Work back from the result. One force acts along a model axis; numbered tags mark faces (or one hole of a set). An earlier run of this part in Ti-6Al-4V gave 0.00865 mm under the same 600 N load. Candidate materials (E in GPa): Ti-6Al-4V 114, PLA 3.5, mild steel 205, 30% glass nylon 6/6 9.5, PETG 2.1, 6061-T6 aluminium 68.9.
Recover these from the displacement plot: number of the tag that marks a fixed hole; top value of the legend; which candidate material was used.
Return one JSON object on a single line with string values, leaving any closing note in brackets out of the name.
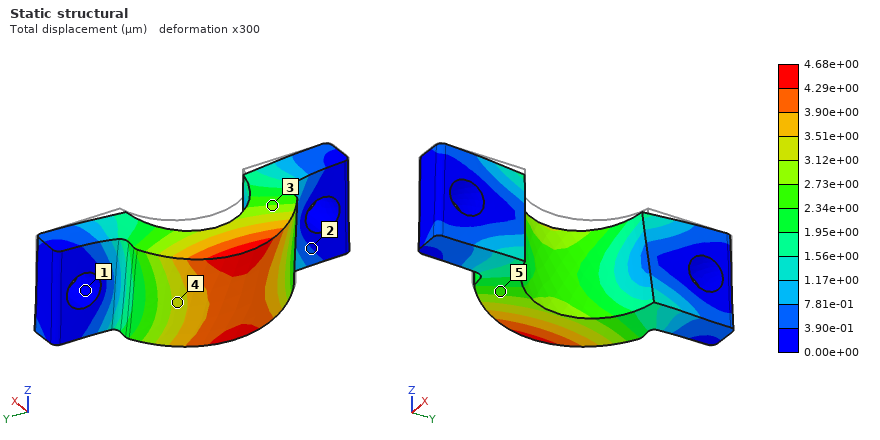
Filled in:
{"number of the tag that marks a fixed hole": "1", "top value of the legend": "4.68e+00 µm", "which candidate material was used": "mild steel"}
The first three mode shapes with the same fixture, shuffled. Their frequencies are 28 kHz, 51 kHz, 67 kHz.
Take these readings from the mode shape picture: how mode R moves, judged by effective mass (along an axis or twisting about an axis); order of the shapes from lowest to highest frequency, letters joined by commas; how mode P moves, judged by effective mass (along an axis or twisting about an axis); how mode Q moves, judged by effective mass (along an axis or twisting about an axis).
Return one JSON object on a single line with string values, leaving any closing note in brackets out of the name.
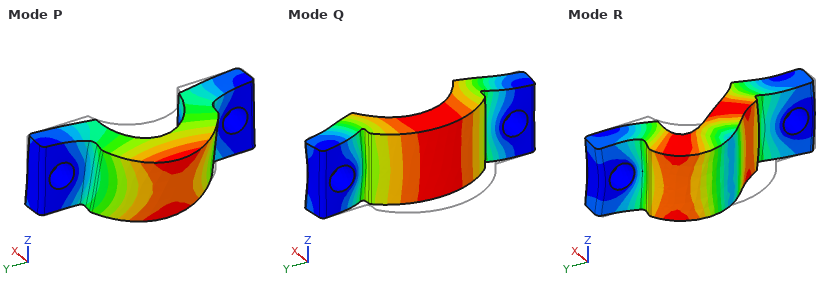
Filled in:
{"how mode R moves, judged by effective mass": "along Y", "order of the shapes from lowest to highest frequency, letters joined by commas": "P, Q, R", "how mode P moves, judged by effective mass": "along Z", "how mode Q moves, judged by effective mass": "along X"}
